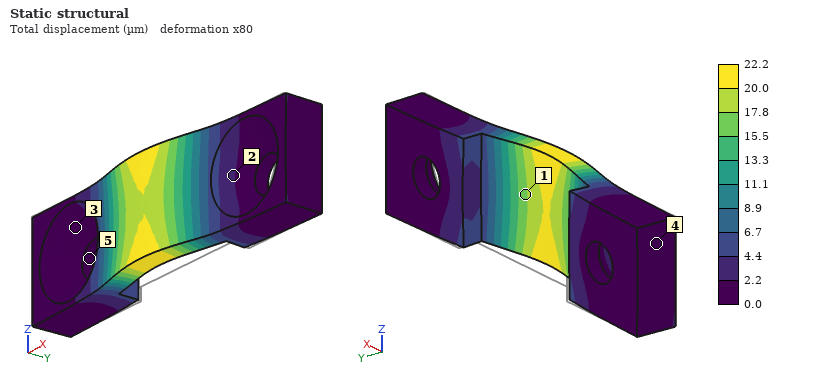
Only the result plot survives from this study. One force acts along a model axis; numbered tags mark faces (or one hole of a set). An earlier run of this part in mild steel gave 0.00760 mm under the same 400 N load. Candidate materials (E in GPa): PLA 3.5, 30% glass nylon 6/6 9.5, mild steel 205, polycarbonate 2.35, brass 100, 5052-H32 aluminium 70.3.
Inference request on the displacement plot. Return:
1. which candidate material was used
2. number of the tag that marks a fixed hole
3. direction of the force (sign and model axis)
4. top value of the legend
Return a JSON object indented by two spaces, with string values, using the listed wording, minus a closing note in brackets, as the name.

{
  "which candidate material was used": "5052-H32 aluminium",
  "number of the tag that marks a fixed hole": "5",
  "direction of the force": "-Y",
  "top value of the legend": "22.2 µm"
}
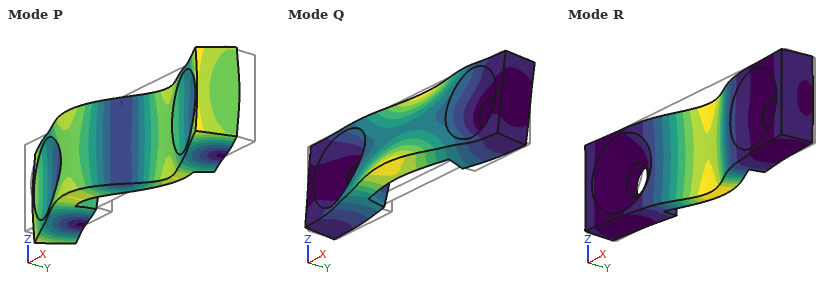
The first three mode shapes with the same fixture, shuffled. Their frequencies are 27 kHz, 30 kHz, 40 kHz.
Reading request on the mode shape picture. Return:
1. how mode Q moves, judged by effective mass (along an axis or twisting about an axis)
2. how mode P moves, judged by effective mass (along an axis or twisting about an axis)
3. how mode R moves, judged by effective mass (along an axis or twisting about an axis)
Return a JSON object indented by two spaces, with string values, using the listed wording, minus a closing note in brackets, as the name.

{
  "how mode Q moves, judged by effective mass": "along Z",
  "how mode P moves, judged by effective mass": "along X",
  "how mode R moves, judged by effective mass": "along Y"
}
